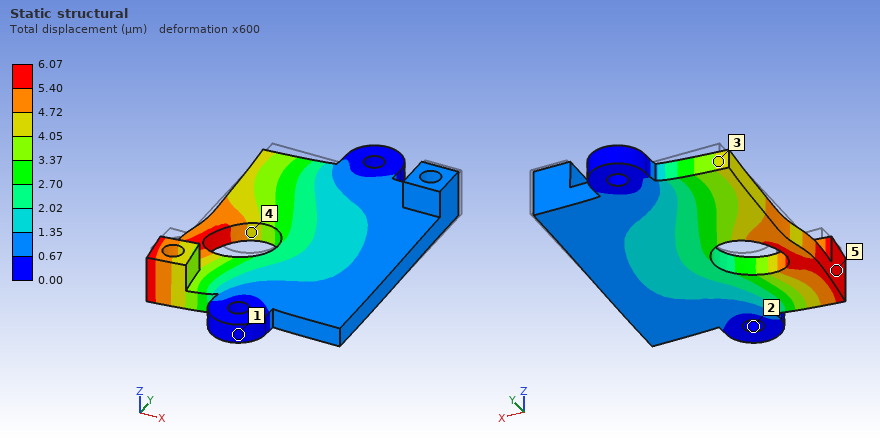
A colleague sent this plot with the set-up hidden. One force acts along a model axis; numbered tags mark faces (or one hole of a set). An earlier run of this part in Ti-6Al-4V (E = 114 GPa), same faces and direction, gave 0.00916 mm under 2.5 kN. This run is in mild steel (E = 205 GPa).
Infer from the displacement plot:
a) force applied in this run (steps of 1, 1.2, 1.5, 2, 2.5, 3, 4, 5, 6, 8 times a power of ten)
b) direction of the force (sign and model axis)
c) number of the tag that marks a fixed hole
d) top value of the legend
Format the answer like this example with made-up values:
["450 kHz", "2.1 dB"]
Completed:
["3 kN", "-Y", "2", "6.07 µm"]
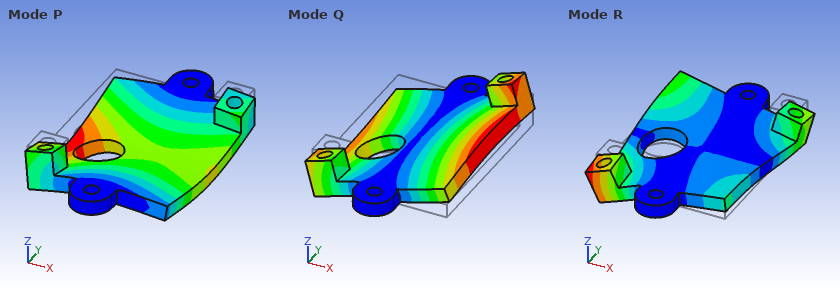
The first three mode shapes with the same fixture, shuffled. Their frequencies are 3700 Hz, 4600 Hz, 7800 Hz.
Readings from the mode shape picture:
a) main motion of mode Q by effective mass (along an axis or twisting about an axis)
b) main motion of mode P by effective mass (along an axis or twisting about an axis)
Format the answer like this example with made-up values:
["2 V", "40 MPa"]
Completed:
["twisting about Y", "along Z"]
